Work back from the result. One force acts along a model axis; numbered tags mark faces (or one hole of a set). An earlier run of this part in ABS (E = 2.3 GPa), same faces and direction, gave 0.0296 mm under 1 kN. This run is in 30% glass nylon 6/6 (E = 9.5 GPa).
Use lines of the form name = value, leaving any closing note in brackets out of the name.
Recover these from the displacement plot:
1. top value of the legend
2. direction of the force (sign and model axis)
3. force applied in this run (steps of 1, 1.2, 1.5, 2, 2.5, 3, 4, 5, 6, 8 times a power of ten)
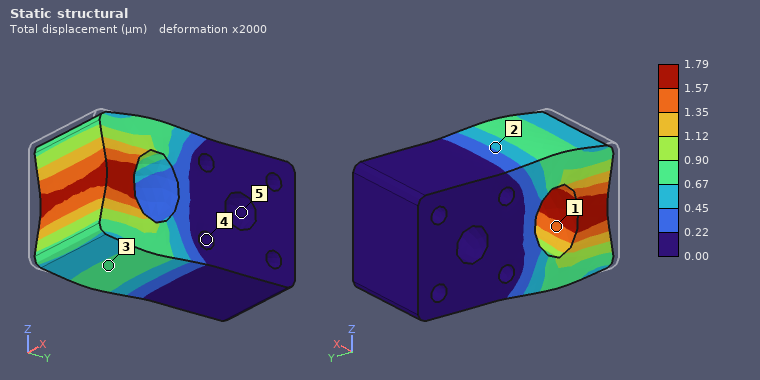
top value of the legend = 1.79 µm
direction of the force = +Y
force applied in this run = 250 N
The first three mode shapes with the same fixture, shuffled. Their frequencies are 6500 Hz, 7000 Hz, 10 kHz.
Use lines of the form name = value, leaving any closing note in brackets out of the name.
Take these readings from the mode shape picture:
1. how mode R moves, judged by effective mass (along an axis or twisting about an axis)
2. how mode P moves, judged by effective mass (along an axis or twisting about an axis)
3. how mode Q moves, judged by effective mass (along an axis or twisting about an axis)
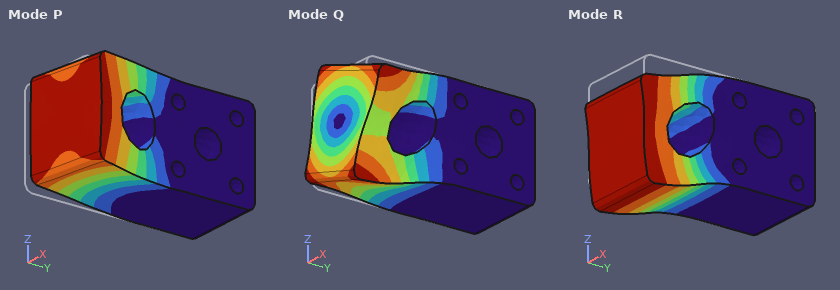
how mode R moves, judged by effective mass = along Z
how mode P moves, judged by effective mass = along X
how mode Q moves, judged by effective mass = twisting about Y
